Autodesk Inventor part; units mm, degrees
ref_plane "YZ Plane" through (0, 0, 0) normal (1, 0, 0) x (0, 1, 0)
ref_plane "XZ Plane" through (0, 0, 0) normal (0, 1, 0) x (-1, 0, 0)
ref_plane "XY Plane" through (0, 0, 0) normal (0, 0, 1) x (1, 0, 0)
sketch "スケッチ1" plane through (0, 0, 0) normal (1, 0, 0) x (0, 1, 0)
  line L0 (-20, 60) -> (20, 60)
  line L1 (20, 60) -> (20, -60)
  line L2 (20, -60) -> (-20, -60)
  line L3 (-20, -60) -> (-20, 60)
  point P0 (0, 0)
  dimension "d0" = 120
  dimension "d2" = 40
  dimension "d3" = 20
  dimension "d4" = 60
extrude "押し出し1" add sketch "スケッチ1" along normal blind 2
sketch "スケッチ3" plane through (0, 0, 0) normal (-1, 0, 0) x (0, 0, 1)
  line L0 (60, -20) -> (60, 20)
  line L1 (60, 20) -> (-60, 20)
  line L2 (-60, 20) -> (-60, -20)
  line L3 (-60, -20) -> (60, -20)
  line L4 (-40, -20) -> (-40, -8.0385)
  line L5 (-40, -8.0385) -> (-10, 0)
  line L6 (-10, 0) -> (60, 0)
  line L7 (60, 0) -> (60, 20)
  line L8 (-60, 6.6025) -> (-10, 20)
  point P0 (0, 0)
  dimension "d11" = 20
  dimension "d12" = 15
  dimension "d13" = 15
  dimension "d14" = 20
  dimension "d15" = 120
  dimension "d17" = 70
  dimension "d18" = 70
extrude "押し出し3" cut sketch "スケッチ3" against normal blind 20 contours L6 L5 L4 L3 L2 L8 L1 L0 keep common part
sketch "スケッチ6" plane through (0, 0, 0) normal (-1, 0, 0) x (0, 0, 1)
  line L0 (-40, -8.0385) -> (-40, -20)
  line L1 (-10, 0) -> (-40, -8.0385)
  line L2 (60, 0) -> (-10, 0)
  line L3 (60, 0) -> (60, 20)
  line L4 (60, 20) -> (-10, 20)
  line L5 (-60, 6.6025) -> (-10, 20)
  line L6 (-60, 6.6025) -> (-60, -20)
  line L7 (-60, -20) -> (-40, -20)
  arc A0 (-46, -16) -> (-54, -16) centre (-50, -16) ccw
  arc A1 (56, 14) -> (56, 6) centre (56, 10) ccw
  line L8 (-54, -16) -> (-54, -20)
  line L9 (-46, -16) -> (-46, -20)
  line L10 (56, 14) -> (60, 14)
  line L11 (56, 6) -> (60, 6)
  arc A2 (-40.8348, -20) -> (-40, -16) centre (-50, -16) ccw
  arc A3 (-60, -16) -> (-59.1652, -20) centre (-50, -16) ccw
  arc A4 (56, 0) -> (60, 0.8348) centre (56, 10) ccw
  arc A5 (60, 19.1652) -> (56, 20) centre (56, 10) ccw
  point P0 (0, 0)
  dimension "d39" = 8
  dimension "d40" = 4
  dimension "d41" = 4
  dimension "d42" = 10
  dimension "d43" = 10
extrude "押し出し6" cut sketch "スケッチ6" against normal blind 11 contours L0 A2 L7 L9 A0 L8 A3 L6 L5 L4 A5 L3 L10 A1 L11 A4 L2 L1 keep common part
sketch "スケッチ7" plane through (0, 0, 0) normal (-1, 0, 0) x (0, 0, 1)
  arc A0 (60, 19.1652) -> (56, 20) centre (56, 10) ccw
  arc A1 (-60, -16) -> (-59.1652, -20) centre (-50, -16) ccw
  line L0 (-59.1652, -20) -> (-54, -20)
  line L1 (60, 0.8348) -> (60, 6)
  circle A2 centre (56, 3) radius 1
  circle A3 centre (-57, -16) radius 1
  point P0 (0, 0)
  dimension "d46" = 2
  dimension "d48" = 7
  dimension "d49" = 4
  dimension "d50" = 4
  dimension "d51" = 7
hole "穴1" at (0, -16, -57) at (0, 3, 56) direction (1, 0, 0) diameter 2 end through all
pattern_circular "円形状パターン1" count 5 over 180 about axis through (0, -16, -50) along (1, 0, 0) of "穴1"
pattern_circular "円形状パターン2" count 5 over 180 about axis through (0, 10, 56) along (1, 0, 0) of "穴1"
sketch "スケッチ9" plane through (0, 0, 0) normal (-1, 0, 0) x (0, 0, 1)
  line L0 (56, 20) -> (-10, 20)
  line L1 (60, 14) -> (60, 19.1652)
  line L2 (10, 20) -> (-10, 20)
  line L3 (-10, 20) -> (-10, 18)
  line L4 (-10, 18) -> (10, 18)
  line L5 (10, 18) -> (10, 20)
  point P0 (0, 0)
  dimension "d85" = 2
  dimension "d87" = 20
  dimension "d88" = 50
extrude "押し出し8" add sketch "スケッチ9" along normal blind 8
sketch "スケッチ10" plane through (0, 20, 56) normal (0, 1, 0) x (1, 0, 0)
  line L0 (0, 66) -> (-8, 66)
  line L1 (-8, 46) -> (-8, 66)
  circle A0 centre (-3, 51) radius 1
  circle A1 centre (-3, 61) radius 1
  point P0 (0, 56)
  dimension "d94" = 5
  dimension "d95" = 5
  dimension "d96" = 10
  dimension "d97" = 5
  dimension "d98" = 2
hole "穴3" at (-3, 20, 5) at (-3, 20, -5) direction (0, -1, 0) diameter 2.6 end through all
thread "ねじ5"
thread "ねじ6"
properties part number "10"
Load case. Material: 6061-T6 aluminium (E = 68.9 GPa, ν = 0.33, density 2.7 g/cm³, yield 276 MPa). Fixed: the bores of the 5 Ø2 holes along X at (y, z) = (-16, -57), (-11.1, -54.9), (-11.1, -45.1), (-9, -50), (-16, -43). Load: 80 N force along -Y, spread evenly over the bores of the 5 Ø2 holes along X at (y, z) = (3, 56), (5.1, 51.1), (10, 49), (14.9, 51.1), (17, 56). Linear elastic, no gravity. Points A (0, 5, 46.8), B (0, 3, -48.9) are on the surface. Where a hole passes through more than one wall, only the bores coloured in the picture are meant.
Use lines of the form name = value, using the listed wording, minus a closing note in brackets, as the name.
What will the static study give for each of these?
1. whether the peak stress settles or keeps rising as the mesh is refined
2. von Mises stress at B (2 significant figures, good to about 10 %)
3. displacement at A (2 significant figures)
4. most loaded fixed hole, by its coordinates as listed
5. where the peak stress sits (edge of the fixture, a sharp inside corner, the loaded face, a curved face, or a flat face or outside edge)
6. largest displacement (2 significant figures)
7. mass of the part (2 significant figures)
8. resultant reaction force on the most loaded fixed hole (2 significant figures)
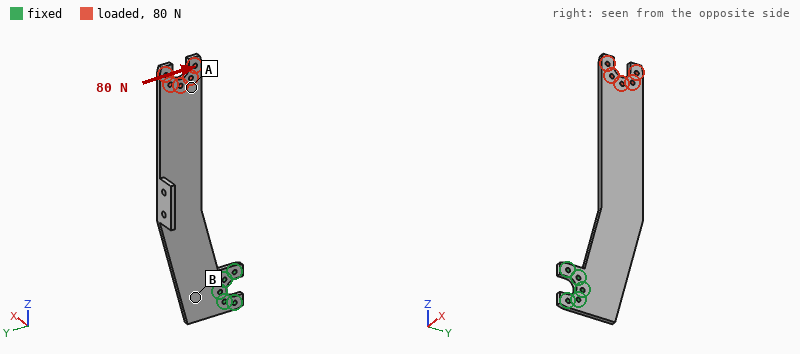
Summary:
whether the peak stress settles or keeps rising as the mesh is refined = keeps rising
von Mises stress at B = 32 MPa
displacement at A = 0.40 mm
most loaded fixed hole, by its coordinates as listed = (-11.1, -45.1)
where the peak stress sits = a sharp inside corner
largest displacement = 0.48 mm
mass of the part = 14 g
resultant reaction force on the most loaded fixed hole = 460 N
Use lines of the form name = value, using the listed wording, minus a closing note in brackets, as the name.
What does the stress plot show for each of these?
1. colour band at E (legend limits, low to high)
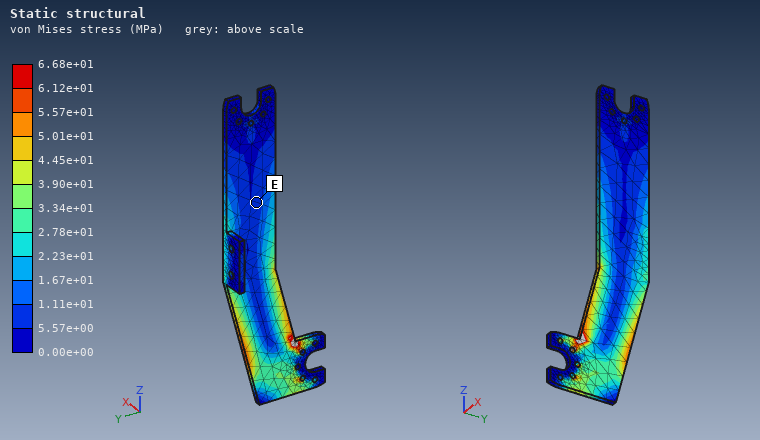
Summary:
colour band at E = 5.57e+00 to 1.11e+01 MPa
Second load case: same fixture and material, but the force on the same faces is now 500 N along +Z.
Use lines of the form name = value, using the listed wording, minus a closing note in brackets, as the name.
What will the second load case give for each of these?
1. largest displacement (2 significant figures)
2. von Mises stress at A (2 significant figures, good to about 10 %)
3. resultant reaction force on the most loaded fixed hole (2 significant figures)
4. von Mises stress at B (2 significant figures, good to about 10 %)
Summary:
largest displacement = 0.27 mm
von Mises stress at A = 12 MPa
resultant reaction force on the most loaded fixed hole = 470 N
von Mises stress at B = 32 MPa
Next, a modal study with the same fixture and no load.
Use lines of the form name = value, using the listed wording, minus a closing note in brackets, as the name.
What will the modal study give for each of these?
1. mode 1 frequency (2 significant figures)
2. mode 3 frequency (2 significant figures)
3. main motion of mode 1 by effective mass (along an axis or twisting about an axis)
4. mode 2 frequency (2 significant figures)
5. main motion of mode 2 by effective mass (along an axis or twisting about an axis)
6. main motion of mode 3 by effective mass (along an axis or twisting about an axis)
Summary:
mode 1 frequency = 140 Hz
mode 3 frequency = 1100 Hz
main motion of mode 1 by effective mass = along X
mode 2 frequency = 760 Hz
main motion of mode 2 by effective mass = along X
main motion of mode 3 by effective mass = along Y
